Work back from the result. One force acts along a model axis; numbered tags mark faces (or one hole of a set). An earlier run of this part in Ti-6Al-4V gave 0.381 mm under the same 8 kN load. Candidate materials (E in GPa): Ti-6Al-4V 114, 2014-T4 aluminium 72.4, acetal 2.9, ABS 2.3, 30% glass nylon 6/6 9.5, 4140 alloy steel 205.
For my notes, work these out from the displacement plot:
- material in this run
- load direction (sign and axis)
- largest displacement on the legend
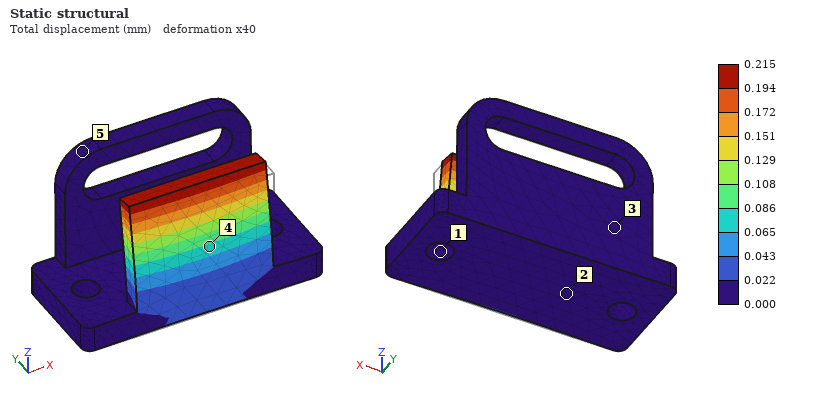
4140 alloy steel
+Y
0.215 mm
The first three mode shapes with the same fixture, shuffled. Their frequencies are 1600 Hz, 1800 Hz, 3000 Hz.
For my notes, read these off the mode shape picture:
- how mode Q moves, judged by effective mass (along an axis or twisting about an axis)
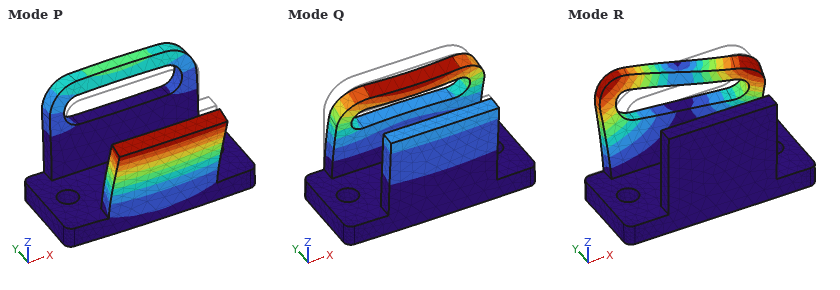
along Y
